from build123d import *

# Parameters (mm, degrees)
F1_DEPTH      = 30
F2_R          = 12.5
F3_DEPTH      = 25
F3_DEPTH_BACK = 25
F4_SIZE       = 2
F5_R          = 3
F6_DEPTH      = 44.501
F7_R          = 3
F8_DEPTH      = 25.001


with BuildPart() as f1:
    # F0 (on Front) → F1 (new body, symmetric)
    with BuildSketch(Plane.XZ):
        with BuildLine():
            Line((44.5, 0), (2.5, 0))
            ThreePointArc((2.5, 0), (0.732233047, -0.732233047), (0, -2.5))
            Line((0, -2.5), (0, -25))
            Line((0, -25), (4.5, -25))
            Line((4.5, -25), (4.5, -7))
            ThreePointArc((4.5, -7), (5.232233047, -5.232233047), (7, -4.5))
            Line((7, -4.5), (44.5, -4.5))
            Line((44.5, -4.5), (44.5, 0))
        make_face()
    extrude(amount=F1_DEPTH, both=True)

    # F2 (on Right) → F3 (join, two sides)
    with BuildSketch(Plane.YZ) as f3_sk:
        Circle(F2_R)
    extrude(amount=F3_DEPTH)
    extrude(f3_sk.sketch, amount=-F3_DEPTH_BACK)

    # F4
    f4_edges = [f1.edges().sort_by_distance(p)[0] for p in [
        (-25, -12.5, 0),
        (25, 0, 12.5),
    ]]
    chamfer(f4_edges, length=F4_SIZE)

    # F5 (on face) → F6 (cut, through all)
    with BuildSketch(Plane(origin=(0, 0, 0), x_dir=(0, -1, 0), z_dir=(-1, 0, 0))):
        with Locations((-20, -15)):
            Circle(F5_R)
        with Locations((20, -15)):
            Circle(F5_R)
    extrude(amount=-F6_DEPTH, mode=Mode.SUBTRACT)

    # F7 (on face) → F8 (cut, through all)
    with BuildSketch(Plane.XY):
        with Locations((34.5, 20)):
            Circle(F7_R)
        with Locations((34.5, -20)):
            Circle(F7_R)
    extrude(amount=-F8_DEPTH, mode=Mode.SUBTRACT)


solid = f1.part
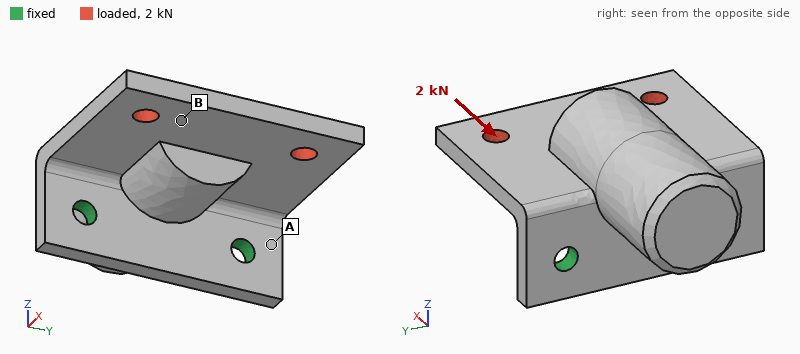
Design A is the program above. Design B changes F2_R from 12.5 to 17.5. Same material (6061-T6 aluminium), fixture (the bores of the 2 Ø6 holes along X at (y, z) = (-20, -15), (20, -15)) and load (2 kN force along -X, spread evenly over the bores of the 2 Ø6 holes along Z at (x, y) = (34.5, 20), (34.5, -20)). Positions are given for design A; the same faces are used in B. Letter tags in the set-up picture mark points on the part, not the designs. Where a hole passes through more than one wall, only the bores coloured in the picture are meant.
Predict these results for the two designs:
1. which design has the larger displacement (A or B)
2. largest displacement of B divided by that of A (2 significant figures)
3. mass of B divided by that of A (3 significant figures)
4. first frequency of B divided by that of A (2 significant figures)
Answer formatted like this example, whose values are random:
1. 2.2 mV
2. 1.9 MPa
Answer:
1. A
2. 0.80
3. 1.56
4. 0.94
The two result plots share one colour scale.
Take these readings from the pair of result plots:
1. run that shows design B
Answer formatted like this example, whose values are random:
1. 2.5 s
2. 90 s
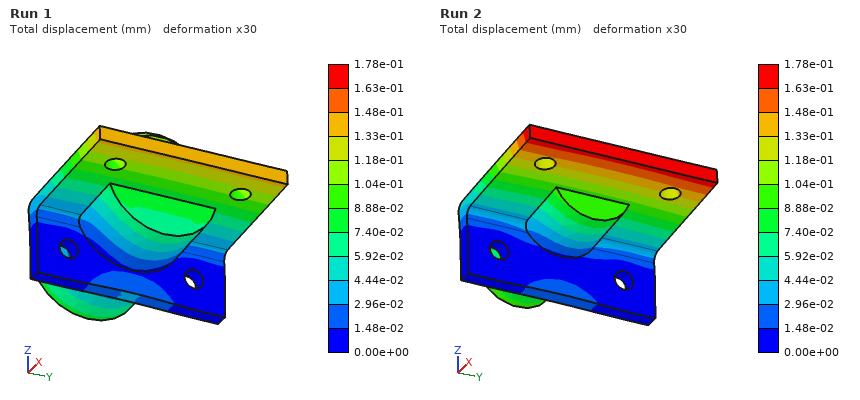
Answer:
1. Run 1
